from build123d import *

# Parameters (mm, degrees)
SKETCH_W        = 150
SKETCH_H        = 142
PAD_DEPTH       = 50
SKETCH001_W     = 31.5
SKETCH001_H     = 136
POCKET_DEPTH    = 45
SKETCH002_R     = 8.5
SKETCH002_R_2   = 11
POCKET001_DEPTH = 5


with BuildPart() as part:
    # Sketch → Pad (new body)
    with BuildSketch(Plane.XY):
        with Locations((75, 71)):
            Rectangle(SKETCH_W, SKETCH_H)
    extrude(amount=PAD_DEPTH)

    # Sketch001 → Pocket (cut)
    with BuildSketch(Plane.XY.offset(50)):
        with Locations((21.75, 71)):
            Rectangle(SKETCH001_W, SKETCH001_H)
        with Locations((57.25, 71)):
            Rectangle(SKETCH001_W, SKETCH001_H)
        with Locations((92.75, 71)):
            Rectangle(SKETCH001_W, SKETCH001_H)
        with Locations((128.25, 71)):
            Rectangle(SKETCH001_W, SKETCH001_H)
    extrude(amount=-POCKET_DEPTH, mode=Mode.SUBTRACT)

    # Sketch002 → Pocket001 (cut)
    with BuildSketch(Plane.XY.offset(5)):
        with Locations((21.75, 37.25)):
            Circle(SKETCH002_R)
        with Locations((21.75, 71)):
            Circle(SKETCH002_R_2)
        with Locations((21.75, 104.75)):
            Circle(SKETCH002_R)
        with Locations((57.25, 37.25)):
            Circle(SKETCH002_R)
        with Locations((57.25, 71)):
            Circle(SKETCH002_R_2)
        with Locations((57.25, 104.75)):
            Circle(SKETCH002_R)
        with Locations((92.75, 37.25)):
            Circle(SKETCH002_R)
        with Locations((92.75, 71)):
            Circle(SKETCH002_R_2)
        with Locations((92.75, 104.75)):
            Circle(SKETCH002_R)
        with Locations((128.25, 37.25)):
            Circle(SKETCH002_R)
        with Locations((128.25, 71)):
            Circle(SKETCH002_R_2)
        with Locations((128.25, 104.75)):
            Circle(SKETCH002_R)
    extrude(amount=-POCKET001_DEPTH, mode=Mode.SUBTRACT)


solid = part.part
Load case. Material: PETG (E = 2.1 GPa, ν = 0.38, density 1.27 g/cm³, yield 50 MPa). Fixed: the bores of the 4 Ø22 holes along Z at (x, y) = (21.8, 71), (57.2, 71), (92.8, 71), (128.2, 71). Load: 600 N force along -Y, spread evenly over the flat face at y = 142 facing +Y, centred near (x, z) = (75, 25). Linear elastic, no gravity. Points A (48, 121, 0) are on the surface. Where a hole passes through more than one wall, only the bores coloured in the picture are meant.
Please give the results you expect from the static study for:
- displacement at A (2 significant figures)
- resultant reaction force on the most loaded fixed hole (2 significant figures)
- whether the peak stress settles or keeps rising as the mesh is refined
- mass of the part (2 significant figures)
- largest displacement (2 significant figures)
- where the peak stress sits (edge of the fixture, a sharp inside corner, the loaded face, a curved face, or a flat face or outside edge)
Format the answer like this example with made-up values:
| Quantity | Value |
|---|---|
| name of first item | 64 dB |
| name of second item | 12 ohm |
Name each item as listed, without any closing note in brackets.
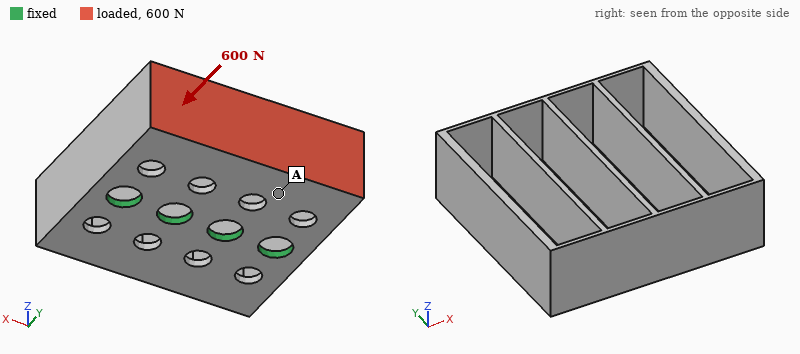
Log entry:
| Quantity | Value |
|---|---|
| displacement at A | 0.17 mm |
| resultant reaction force on the most loaded fixed hole | 160 N |
| whether the peak stress settles or keeps rising as the mesh is refined | keeps rising |
| mass of the part | 350 g |
| largest displacement | 0.36 mm |
| where the peak stress sits | edge of the fixture |
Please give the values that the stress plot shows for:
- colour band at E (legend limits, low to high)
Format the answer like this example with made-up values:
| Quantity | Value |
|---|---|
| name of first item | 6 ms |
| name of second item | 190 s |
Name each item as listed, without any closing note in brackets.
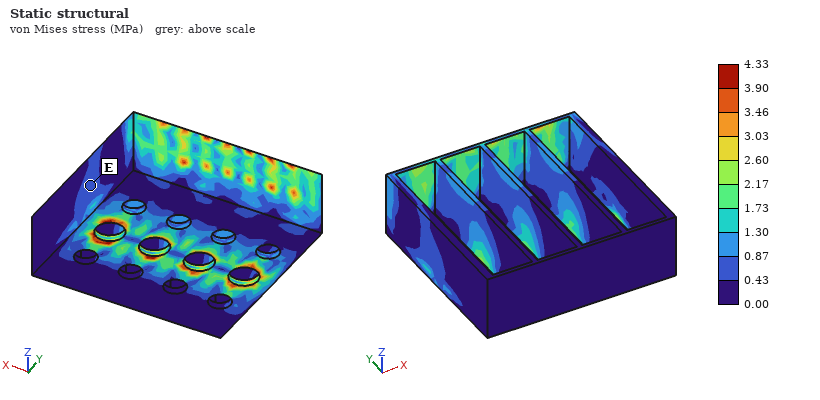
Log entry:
| Quantity | Value |
|---|---|
| colour band at E | 0.43 to 0.87 MPa |
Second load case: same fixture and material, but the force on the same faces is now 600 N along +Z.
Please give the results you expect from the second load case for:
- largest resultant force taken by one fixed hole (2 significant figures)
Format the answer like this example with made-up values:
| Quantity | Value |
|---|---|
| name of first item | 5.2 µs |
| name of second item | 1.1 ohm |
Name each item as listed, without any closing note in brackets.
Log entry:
| Quantity | Value |
|---|---|
| largest resultant force taken by one fixed hole | 180 N |
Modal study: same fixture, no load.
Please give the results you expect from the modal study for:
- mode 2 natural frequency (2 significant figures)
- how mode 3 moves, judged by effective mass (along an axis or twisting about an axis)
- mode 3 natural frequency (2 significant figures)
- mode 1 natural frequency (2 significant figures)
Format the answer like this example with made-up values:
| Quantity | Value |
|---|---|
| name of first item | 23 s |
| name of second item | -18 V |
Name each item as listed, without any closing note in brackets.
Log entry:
| Quantity | Value |
|---|---|
| mode 2 natural frequency | 330 Hz |
| how mode 3 moves, judged by effective mass | along X |
| mode 3 natural frequency | 510 Hz |
| mode 1 natural frequency | 290 Hz |
